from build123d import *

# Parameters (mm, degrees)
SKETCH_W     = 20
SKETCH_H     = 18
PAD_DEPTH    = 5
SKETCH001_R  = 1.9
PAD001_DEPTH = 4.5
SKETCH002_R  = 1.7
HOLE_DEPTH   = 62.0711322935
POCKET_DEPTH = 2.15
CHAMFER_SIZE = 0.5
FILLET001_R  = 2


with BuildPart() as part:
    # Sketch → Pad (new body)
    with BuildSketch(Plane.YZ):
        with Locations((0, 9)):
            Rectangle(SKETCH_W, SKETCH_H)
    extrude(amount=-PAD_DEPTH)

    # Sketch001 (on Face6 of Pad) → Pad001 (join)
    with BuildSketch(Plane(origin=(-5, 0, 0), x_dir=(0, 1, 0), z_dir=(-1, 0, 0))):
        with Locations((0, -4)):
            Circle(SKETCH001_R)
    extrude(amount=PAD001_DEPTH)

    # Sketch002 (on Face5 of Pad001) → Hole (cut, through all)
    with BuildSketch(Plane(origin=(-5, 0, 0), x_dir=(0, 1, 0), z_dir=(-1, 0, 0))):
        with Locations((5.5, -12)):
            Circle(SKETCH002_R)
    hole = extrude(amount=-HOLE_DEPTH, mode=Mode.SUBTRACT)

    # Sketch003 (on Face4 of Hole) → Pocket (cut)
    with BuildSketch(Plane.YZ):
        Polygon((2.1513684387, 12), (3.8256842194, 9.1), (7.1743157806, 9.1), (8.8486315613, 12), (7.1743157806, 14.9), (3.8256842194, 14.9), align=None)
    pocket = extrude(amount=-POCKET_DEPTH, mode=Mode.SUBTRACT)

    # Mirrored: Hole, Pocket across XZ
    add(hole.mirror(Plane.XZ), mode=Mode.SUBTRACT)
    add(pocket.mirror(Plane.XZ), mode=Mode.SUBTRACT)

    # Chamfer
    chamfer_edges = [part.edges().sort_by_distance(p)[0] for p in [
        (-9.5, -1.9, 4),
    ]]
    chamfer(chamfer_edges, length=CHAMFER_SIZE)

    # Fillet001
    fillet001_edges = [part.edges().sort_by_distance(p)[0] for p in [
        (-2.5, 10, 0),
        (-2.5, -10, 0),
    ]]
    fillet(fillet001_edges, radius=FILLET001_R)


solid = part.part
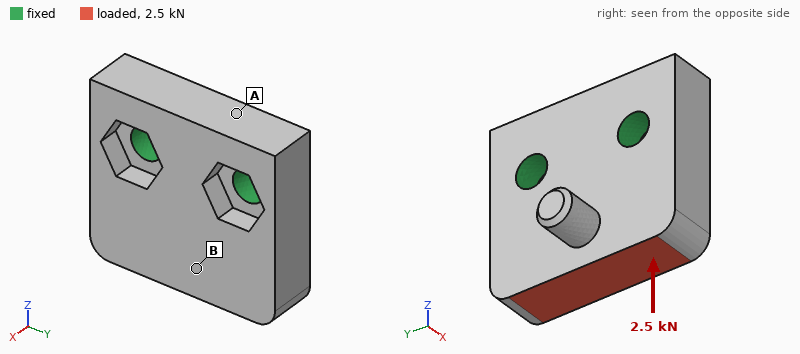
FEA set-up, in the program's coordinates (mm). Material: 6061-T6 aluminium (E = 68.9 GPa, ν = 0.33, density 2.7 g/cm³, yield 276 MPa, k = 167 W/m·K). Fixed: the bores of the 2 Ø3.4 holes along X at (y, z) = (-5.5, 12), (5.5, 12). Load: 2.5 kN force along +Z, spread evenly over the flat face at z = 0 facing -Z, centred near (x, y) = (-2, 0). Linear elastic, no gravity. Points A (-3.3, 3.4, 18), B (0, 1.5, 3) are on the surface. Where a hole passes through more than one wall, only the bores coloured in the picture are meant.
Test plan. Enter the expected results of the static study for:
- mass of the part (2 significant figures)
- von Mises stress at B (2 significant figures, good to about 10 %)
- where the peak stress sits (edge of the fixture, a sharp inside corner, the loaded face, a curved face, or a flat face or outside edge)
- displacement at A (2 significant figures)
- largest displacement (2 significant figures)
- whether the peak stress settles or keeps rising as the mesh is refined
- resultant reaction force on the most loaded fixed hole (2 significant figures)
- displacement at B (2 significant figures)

4.5 g
32 MPa
edge of the fixture
3.9 µm
18 µm
keeps rising
1.3 kN
14 µm
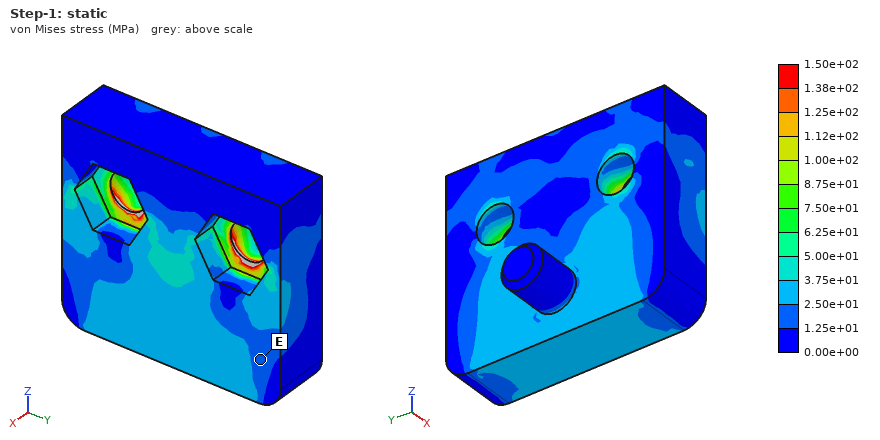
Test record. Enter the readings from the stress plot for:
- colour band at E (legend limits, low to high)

1.25e+01 to 2.50e+01 MPa
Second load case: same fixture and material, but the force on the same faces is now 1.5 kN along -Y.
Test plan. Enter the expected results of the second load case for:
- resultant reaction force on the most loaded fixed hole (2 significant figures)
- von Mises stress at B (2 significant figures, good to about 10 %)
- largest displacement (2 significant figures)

1.5 kN
34 MPa
17 µm
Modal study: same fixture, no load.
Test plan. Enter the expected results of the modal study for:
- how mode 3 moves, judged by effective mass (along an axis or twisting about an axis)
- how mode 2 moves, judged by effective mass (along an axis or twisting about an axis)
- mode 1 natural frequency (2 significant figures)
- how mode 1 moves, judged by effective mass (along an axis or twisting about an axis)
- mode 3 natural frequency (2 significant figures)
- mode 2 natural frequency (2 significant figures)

along Y
twisting about Z
18 kHz
along X
43 kHz
32 kHz
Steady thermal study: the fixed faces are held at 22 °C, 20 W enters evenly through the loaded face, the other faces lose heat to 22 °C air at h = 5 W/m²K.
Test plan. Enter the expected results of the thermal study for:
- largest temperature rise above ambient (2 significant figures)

17 K
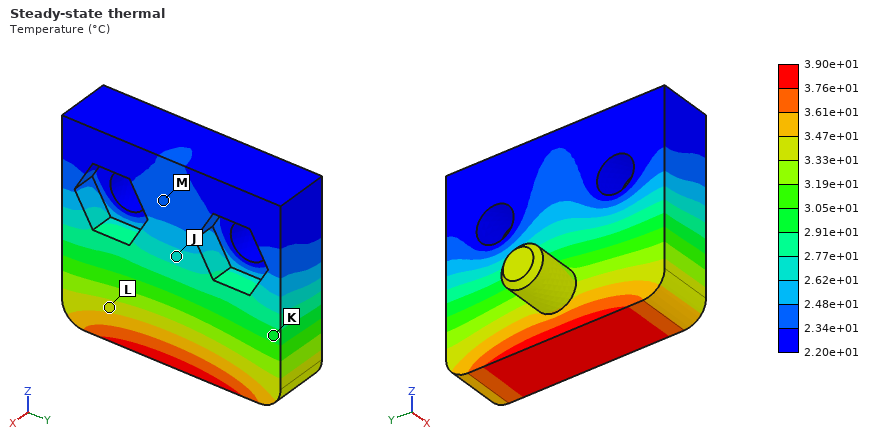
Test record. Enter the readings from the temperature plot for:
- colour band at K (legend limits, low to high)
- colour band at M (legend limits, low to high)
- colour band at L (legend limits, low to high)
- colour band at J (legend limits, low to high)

2.91e+01 to 3.05e+01 °C
2.34e+01 to 2.48e+01 °C
3.33e+01 to 3.47e+01 °C
2.62e+01 to 2.77e+01 °C
